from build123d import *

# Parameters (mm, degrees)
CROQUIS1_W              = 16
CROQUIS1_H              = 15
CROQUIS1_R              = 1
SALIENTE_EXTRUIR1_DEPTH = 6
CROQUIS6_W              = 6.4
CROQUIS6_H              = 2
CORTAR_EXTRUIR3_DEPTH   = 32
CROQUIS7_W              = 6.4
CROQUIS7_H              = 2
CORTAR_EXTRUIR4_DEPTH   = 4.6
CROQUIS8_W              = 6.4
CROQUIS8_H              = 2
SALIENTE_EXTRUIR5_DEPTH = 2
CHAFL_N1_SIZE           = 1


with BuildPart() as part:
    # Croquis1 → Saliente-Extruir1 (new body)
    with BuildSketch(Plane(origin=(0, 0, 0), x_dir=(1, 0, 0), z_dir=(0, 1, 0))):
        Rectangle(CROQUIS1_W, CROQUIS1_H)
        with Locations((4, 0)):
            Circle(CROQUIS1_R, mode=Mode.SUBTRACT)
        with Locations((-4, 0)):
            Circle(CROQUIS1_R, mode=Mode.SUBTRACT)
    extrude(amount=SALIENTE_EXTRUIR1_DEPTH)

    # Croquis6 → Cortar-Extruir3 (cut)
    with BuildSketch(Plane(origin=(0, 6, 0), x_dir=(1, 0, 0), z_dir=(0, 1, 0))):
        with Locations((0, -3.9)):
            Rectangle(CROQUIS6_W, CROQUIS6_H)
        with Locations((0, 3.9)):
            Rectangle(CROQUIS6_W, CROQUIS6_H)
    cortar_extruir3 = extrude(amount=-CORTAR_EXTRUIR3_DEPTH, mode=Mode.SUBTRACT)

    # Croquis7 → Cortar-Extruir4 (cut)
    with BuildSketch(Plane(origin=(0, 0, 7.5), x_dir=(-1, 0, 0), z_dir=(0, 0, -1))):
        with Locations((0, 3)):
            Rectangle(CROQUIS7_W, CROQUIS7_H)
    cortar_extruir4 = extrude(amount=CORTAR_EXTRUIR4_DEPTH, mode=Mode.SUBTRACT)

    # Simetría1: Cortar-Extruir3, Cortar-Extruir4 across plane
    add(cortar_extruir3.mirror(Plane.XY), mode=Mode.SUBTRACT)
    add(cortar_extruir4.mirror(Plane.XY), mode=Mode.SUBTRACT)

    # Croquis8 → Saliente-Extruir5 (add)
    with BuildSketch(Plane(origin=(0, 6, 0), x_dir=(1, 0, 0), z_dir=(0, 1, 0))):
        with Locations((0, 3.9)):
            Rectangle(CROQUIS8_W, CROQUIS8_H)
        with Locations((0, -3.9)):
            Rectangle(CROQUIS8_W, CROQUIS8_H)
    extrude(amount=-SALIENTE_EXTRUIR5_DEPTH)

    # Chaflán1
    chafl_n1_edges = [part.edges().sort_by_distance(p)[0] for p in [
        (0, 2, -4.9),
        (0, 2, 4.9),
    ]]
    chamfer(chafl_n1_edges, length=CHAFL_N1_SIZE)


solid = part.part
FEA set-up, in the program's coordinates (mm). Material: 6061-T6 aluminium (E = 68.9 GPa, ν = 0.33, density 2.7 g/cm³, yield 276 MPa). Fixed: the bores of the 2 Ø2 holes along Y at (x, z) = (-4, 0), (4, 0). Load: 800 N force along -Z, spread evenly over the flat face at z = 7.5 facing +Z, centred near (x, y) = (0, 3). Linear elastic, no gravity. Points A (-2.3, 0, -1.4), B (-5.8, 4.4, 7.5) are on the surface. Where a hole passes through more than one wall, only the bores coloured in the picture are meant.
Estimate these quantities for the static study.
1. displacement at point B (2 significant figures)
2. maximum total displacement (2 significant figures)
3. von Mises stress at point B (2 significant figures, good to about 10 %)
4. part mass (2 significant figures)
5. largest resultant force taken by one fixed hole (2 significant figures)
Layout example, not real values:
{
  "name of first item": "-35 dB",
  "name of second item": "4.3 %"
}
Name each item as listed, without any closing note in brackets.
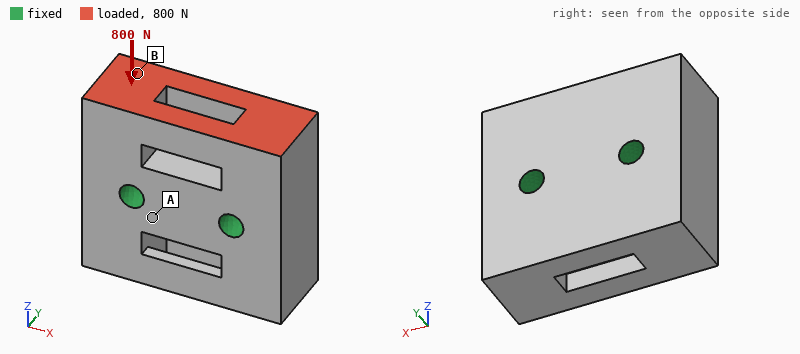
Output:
{
  "displacement at point B": "1.3 µm",
  "maximum total displacement": "4.2 µm",
  "von Mises stress at point B": "11 MPa",
  "part mass": "3.3 g",
  "largest resultant force taken by one fixed hole": "400 N"
}
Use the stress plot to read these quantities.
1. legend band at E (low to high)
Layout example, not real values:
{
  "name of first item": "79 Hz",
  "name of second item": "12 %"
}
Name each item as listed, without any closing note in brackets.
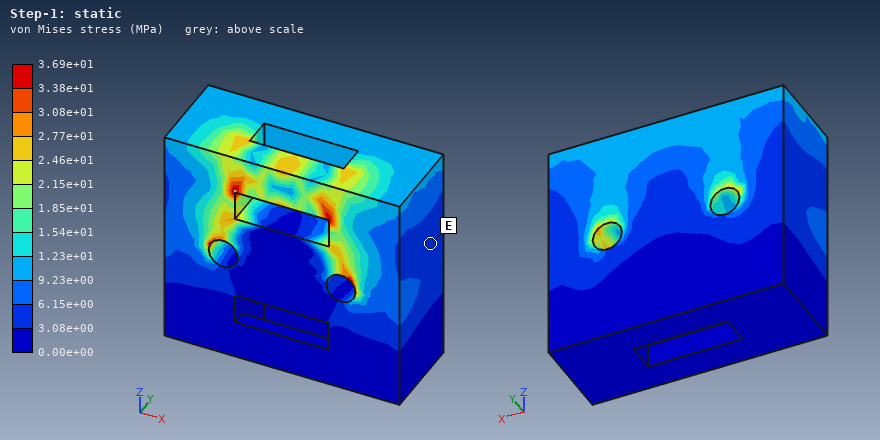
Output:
{
  "legend band at E": "3.08e+00 to 6.15e+00 MPa"
}
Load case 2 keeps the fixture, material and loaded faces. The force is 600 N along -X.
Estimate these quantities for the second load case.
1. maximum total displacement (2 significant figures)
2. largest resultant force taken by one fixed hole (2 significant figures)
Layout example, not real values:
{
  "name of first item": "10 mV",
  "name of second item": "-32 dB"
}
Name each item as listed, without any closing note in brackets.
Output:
{
  "maximum total displacement": "8.1 µm",
  "largest resultant force taken by one fixed hole": "510 N"
}
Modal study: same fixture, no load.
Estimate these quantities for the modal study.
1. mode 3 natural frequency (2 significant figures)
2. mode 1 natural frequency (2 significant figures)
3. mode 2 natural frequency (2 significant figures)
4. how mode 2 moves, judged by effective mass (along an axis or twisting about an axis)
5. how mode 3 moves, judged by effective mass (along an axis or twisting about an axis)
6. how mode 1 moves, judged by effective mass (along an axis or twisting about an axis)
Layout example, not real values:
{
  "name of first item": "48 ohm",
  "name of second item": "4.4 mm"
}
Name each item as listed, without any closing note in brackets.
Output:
{
  "mode 3 natural frequency": "62 kHz",
  "mode 1 natural frequency": "53 kHz",
  "mode 2 natural frequency": "56 kHz",
  "how mode 2 moves, judged by effective mass": "twisting about Y",
  "how mode 3 moves, judged by effective mass": "along Y",
  "how mode 1 moves, judged by effective mass": "twisting about X"
}
